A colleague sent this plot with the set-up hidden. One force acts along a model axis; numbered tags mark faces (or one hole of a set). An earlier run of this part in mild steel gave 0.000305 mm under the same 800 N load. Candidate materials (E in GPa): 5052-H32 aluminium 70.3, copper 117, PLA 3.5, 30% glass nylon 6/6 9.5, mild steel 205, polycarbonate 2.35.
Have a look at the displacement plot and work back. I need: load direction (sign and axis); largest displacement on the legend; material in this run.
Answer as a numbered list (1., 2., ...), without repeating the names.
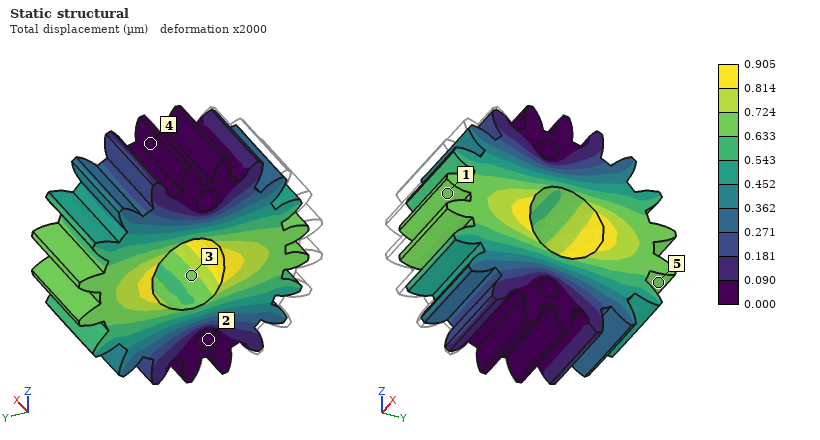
1. +Y
2. 0.905 µm
3. 5052-H32 aluminium
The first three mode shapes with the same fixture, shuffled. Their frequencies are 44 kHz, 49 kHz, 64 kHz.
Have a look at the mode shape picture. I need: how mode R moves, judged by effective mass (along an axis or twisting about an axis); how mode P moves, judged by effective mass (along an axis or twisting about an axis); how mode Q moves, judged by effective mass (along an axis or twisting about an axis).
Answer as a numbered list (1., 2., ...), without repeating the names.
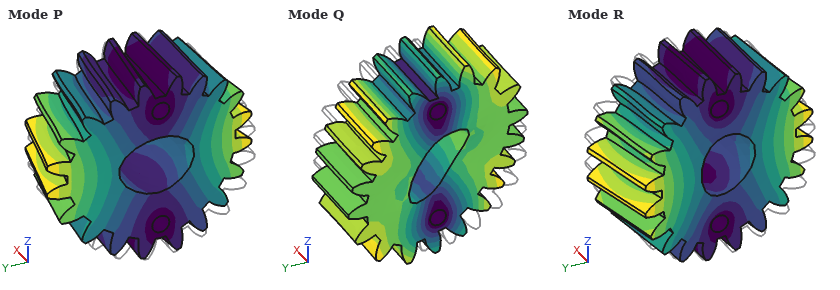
1. twisting about Z
2. along X
3. twisting about X
